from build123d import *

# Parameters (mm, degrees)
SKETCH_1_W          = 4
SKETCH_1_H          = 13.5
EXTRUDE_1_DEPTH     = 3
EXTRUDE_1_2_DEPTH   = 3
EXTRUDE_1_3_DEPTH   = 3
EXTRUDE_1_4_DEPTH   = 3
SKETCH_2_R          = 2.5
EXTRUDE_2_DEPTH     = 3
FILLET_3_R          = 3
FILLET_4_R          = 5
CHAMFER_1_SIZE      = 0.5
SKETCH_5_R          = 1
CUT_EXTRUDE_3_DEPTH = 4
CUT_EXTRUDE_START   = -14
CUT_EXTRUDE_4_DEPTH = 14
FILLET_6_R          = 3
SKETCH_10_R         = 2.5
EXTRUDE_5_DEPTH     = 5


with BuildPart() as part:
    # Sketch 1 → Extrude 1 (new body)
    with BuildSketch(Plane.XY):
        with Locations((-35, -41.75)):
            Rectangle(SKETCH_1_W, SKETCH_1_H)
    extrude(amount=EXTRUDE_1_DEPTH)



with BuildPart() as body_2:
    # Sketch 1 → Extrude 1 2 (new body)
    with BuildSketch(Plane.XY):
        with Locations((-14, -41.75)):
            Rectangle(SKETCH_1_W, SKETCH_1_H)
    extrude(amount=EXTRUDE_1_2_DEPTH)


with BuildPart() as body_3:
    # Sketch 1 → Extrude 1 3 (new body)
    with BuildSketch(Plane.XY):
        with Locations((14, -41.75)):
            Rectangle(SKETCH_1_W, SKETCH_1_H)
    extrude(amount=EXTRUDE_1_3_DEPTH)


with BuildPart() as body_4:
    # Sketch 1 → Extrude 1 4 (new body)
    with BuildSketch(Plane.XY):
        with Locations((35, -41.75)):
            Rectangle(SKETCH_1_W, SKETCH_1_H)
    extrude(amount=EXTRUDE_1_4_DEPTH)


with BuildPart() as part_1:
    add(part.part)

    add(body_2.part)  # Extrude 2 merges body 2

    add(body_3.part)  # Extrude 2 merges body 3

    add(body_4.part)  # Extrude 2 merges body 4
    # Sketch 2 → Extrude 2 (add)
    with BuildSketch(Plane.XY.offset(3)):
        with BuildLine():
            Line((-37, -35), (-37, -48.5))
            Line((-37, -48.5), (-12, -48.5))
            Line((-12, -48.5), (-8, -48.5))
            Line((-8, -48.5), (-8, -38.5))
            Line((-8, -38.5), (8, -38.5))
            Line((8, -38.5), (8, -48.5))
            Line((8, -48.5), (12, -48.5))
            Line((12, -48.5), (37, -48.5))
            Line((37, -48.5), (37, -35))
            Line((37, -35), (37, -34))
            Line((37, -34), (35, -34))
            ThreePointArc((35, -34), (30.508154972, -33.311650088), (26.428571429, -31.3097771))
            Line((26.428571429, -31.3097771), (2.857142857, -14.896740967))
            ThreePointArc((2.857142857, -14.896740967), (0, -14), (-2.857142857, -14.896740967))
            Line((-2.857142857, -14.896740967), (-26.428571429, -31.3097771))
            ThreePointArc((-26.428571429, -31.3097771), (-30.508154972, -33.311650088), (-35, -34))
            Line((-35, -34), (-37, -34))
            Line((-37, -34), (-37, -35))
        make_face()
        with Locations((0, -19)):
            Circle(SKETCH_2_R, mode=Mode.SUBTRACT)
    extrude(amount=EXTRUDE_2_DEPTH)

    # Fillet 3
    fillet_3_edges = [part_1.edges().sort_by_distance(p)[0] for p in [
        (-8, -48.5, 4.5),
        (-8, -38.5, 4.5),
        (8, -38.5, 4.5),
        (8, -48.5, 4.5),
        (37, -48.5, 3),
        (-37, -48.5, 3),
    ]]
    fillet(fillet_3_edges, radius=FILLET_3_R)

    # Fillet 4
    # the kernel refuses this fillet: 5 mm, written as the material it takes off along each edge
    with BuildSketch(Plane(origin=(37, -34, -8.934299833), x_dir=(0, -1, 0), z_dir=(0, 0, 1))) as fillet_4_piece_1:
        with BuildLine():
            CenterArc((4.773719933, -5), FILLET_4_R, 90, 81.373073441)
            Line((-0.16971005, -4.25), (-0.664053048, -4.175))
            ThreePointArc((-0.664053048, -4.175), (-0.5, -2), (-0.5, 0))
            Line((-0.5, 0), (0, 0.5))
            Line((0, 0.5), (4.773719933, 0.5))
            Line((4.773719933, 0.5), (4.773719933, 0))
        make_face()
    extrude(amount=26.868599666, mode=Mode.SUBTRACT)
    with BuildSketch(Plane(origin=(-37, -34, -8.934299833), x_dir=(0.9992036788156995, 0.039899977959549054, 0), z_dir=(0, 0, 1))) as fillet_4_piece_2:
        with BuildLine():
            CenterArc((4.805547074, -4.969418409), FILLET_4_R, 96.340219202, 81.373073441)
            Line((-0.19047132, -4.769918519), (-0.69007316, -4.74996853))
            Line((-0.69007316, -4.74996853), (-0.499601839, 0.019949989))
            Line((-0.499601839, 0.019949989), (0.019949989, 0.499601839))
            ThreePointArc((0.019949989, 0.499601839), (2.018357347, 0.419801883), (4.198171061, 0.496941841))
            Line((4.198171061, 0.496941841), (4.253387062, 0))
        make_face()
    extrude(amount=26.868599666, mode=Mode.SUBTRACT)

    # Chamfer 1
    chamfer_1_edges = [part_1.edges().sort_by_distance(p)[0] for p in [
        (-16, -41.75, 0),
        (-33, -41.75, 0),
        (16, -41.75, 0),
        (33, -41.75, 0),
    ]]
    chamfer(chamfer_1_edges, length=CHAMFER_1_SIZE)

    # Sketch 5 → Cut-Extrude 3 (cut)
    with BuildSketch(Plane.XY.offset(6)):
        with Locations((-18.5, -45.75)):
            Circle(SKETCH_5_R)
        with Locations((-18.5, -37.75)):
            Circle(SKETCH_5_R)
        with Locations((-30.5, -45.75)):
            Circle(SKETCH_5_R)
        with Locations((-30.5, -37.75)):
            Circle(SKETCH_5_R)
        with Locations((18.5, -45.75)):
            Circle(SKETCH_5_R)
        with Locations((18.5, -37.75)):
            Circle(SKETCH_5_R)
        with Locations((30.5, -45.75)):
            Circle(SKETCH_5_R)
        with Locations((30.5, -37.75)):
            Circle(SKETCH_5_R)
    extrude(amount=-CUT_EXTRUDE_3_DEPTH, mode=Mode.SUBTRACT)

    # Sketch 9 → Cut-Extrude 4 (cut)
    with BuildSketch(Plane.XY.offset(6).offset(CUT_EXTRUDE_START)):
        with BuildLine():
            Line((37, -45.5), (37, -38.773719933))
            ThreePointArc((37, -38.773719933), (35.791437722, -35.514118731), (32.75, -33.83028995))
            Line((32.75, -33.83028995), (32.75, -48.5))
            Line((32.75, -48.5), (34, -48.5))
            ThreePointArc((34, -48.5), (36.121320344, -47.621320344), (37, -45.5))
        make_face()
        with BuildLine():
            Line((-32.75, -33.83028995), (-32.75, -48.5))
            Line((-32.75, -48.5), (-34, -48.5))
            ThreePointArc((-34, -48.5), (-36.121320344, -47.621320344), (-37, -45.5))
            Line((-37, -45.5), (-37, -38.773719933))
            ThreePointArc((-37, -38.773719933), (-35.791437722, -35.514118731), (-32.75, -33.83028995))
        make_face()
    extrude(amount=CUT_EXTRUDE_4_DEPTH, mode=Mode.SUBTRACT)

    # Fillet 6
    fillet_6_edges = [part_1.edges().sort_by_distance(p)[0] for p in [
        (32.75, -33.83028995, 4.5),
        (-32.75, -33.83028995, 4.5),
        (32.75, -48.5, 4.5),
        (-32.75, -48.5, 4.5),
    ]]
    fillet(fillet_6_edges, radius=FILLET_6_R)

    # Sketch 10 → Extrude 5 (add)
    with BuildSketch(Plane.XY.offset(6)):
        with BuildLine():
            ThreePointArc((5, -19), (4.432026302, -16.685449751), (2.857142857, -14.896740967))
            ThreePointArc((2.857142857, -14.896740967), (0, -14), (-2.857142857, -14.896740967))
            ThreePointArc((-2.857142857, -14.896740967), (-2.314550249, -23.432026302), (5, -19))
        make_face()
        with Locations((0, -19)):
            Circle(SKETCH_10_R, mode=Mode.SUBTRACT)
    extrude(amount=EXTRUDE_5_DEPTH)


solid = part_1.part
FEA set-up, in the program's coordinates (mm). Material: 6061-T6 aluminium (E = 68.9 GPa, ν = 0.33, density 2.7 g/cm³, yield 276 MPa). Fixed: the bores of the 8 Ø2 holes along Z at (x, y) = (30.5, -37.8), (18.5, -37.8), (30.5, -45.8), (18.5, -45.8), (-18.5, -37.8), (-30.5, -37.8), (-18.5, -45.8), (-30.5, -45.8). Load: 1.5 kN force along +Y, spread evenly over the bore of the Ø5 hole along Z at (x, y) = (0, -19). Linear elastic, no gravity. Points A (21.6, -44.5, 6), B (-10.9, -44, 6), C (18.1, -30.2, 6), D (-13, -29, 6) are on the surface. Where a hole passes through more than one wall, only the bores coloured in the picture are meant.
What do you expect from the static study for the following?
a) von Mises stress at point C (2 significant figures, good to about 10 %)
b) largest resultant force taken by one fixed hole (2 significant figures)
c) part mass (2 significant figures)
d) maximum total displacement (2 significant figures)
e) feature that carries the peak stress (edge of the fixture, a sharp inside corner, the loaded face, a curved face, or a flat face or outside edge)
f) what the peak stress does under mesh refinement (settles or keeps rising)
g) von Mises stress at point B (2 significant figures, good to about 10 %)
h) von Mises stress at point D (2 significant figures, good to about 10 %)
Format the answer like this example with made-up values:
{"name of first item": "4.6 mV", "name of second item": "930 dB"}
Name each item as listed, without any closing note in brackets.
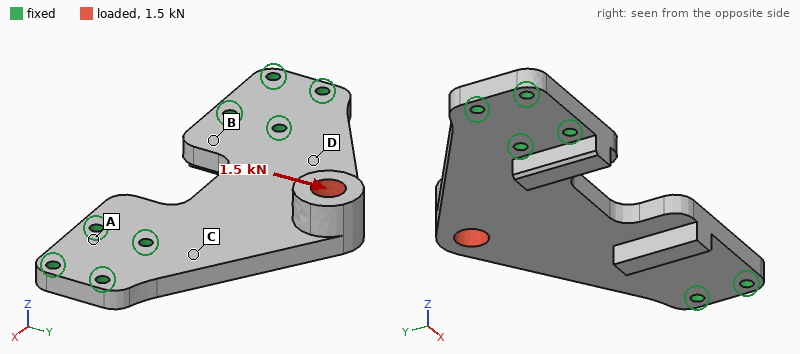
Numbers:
{"von Mises stress at point C": "68 MPa", "largest resultant force taken by one fixed hole": "550 N", "part mass": "13 g", "maximum total displacement": "0.25 mm", "feature that carries the peak stress": "edge of the fixture", "what the peak stress does under mesh refinement": "keeps rising", "von Mises stress at point B": "20 MPa", "von Mises stress at point D": "78 MPa"}
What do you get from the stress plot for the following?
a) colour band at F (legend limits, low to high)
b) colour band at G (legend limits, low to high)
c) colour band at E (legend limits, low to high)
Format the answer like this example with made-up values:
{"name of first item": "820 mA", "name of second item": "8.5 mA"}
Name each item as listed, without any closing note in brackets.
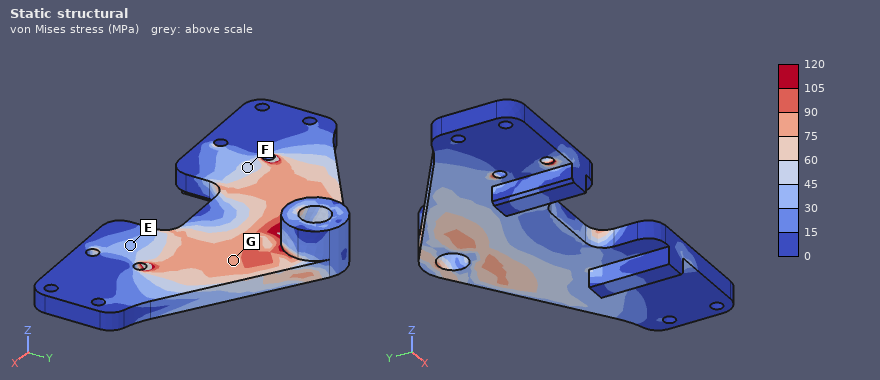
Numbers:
{"colour band at F": "45 to 60 MPa", "colour band at G": "75 to 90 MPa", "colour band at E": "30 to 45 MPa"}
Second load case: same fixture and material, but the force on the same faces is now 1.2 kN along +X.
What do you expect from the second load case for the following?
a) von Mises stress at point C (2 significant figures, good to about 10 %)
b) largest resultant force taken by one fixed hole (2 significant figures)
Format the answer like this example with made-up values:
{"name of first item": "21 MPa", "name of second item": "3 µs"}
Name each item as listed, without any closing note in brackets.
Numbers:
{"von Mises stress at point C": "13 MPa", "largest resultant force taken by one fixed hole": "450 N"}
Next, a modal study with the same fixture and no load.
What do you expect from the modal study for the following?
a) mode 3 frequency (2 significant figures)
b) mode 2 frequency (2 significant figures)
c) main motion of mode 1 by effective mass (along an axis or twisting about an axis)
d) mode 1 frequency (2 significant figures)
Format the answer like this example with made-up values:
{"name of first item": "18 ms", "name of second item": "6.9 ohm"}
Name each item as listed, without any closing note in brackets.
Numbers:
{"mode 3 frequency": "13 kHz", "mode 2 frequency": "13 kHz", "main motion of mode 1 by effective mass": "along Z", "mode 1 frequency": "4400 Hz"}
